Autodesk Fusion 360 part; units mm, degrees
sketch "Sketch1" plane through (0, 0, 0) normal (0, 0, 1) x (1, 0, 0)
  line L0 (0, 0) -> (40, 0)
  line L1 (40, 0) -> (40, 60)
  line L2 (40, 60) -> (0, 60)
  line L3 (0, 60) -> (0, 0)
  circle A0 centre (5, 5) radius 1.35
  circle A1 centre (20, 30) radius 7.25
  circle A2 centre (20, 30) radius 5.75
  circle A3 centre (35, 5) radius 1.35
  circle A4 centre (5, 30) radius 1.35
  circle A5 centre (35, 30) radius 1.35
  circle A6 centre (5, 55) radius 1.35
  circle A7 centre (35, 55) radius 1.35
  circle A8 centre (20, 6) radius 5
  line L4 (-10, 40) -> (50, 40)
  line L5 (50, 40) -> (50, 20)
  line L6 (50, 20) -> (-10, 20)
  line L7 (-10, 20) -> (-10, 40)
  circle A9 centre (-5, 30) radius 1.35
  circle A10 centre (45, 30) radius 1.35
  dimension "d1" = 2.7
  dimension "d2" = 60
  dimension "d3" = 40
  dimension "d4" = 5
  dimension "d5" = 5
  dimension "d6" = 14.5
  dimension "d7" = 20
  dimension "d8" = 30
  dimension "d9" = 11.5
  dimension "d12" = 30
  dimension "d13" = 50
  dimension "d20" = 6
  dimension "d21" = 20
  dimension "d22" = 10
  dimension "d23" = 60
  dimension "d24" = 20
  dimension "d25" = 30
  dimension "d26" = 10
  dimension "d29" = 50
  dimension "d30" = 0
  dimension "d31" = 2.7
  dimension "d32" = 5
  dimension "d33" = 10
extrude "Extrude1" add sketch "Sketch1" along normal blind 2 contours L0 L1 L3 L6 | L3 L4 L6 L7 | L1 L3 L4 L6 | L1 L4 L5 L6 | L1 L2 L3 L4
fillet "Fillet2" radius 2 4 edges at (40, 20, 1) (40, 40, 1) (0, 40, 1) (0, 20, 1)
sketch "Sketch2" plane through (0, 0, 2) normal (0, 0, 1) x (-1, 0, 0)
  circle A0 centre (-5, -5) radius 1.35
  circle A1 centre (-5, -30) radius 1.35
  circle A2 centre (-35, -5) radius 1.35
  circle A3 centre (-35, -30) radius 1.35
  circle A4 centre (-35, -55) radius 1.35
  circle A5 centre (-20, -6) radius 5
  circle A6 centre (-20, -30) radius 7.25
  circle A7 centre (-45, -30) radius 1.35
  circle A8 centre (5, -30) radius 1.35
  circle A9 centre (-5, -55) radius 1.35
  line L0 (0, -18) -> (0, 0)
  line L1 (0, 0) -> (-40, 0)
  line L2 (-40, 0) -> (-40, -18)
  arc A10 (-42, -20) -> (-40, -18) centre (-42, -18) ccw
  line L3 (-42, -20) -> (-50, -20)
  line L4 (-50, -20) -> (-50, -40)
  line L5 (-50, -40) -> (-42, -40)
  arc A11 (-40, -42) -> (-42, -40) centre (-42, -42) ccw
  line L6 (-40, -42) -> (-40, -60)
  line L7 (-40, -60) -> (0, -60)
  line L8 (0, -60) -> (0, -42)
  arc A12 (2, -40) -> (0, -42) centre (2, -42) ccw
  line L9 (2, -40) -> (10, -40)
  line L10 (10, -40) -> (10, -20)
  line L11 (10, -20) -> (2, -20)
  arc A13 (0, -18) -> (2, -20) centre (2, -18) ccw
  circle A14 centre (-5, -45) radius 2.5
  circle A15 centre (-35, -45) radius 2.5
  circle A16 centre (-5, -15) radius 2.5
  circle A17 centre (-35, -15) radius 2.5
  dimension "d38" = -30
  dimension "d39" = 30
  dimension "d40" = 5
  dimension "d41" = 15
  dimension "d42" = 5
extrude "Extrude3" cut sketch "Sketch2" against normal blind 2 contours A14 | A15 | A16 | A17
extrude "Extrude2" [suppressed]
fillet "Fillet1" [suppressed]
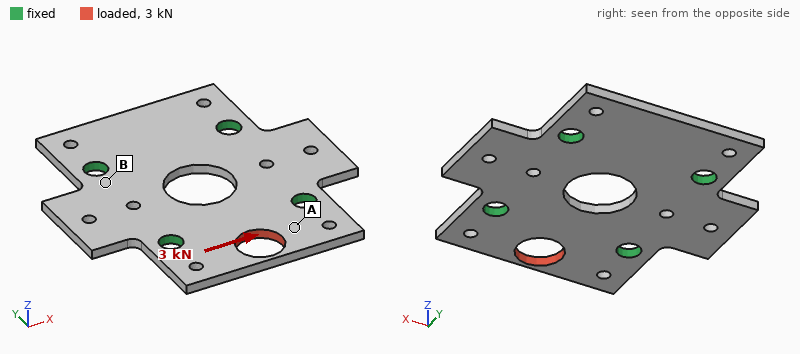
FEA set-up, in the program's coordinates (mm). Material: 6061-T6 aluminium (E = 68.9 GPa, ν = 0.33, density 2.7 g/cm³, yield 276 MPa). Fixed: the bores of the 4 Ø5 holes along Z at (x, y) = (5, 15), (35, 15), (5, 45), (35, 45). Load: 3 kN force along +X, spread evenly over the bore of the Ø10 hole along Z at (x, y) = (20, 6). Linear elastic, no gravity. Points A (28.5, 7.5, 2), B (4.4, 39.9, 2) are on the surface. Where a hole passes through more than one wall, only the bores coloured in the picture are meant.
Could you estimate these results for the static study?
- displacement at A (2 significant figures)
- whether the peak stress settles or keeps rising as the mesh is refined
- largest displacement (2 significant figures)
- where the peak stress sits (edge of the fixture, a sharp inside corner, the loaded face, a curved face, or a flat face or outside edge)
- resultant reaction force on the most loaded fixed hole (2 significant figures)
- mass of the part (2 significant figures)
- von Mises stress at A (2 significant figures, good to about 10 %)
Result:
16 µm
keeps rising
41 µm
a sharp inside corner
1.6 kN
13 g
74 MPa
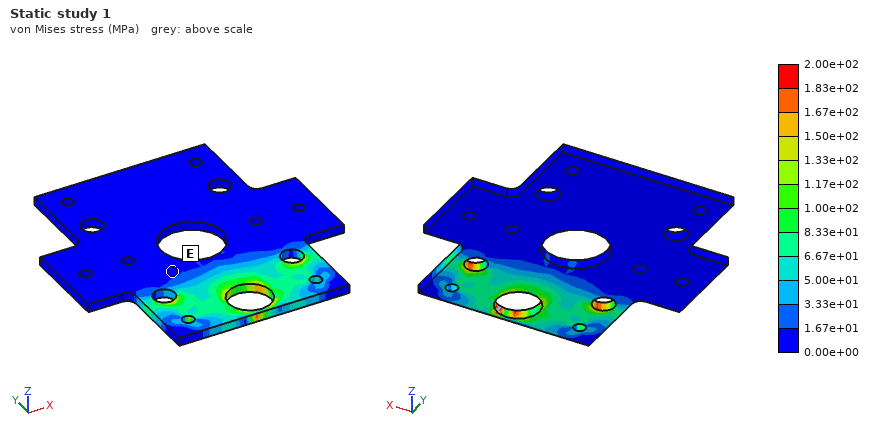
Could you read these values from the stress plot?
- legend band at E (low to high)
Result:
0.00e+00 to 1.67e+01 MPa
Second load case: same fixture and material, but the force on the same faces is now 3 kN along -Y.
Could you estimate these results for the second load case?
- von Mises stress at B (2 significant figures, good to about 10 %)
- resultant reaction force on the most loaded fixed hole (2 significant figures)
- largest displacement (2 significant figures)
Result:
17 MPa
1.4 kN
59 µm
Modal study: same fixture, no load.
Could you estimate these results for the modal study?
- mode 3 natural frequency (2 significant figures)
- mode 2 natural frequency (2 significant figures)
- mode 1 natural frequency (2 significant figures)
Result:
7100 Hz
6200 Hz
6100 Hz
